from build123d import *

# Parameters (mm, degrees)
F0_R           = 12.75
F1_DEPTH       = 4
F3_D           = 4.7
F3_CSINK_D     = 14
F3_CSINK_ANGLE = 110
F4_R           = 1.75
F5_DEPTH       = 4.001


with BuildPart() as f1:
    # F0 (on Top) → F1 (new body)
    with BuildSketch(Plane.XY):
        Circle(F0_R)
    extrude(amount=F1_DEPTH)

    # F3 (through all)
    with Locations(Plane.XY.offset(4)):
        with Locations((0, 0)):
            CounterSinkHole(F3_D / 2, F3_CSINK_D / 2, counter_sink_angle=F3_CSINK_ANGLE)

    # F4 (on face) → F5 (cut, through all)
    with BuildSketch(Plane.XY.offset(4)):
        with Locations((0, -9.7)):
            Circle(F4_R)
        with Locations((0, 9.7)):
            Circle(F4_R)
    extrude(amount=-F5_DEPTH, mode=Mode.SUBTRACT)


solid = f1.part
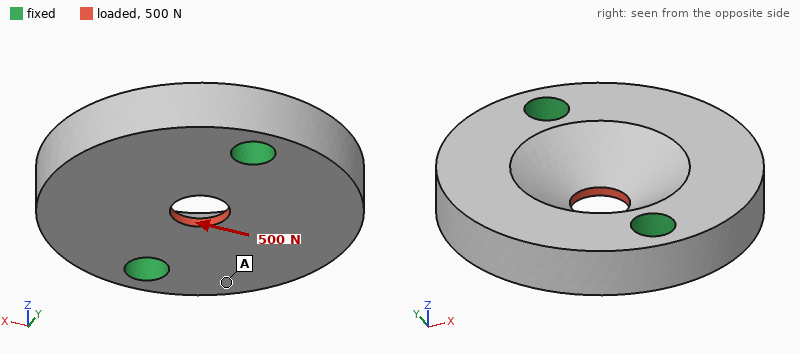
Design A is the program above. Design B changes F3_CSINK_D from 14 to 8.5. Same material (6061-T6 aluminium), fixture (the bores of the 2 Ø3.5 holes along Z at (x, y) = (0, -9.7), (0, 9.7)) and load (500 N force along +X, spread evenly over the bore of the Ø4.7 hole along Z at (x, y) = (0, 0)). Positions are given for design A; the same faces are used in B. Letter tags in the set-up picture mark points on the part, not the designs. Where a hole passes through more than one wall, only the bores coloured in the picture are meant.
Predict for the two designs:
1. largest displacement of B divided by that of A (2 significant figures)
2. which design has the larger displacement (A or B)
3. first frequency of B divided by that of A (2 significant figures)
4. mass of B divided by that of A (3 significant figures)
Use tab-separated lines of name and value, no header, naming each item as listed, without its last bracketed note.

largest displacement of B divided by that of A	0.48
which design has the larger displacement	A
first frequency of B divided by that of A	1.0
mass of B divided by that of A	1.09
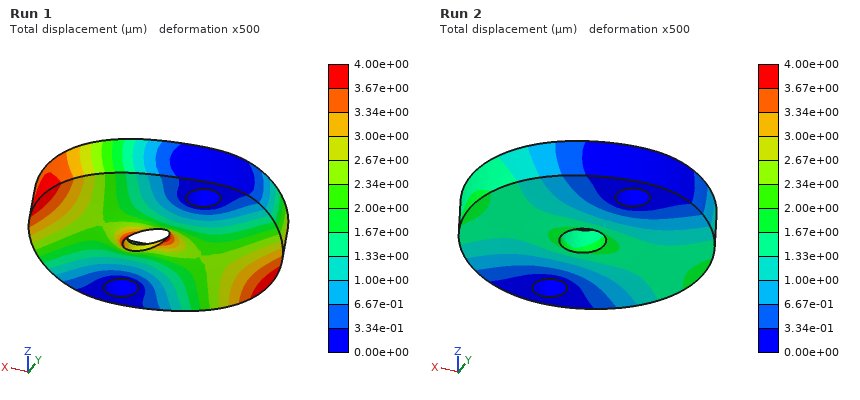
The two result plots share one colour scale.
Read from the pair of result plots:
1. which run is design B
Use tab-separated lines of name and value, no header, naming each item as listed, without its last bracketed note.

which run is design B	Run 2
